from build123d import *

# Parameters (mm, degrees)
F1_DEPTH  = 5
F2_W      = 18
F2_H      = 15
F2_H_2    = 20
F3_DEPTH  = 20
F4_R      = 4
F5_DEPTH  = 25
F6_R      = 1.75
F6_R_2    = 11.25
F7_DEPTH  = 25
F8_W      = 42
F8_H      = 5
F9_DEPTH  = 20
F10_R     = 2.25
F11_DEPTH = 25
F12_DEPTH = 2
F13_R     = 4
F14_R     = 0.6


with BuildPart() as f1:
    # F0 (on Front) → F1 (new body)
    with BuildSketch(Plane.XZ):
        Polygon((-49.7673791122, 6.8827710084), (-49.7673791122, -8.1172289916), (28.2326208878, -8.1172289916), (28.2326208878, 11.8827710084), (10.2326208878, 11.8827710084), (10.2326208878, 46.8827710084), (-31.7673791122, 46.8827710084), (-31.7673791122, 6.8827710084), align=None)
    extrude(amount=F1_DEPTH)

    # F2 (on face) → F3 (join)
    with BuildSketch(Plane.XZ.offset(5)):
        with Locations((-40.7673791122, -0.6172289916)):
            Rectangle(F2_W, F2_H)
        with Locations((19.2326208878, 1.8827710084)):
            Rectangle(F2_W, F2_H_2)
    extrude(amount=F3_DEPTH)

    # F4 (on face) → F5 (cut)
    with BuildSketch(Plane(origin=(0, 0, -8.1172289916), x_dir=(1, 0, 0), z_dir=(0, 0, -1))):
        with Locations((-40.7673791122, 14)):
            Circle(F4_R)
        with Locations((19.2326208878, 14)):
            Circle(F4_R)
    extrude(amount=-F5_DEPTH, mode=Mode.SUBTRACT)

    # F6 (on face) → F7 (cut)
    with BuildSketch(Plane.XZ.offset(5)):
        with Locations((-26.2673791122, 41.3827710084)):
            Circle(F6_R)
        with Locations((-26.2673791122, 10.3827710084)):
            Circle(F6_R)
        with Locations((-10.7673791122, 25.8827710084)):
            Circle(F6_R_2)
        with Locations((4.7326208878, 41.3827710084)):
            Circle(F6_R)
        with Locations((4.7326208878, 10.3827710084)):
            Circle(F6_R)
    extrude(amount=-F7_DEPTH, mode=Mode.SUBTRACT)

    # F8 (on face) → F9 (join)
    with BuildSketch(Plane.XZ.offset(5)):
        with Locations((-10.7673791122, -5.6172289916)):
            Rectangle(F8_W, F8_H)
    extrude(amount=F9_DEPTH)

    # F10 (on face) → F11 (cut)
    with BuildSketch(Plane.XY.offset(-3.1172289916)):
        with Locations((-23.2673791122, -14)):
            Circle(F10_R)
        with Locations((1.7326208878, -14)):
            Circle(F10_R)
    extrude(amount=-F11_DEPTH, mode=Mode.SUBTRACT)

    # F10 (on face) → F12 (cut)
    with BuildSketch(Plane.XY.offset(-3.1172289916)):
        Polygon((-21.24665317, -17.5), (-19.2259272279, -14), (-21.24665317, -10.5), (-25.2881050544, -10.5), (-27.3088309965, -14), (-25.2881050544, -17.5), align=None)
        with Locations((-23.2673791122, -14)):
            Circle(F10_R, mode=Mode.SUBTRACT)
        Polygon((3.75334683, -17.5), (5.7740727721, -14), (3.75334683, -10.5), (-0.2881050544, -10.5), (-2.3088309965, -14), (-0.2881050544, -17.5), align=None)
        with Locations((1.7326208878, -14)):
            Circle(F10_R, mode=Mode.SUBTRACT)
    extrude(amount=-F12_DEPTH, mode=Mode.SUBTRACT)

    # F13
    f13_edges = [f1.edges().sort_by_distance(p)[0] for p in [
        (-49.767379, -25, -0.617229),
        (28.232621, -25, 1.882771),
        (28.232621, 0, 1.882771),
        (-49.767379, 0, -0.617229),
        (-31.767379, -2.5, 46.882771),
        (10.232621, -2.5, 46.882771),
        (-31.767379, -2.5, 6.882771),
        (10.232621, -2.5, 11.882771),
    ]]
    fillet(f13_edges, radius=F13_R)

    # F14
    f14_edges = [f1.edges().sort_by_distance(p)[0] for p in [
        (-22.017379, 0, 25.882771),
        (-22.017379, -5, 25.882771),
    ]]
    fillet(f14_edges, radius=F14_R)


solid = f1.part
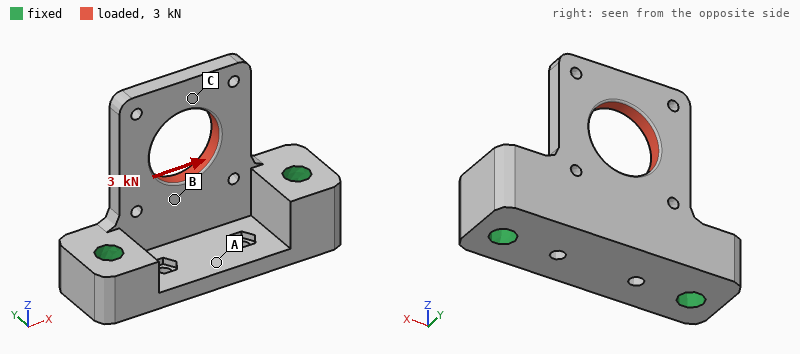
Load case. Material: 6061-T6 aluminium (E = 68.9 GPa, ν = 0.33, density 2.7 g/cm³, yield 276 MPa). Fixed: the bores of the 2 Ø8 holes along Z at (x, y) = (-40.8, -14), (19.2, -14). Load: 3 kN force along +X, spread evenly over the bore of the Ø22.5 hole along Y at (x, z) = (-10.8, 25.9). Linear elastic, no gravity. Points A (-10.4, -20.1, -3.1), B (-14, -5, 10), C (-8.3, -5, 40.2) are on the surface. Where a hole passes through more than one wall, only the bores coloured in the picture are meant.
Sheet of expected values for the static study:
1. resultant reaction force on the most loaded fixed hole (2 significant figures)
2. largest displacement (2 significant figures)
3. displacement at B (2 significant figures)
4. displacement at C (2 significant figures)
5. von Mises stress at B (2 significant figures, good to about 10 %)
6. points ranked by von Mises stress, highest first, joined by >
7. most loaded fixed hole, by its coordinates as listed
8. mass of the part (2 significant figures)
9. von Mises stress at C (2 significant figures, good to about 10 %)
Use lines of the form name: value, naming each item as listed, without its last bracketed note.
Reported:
resultant reaction force on the most loaded fixed hole: 2.3 kN
largest displacement: 74 µm
displacement at B: 11 µm
displacement at C: 67 µm
von Mises stress at B: 37 MPa
points ranked by von Mises stress, highest first, joined by >: B > C > A
most loaded fixed hole, by its coordinates as listed: (19.2, -14)
mass of the part: 73 g
von Mises stress at C: 20 MPa
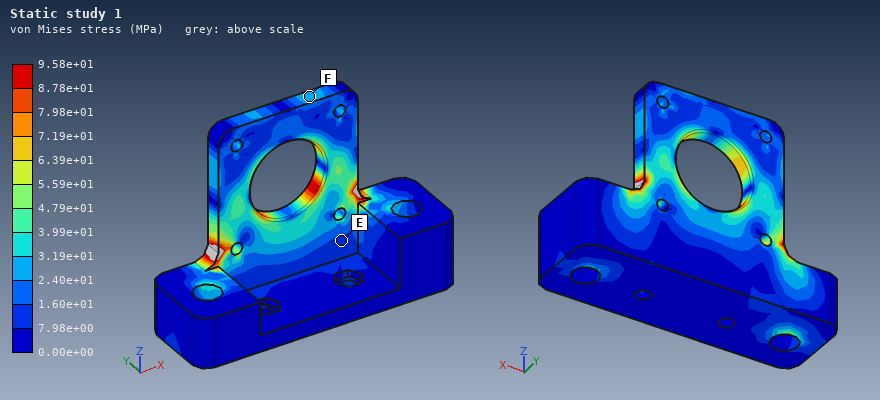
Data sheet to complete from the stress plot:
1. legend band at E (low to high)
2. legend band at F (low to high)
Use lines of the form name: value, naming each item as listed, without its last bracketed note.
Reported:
legend band at E: 7.98e+00 to 1.60e+01 MPa
legend band at F: 2.40e+01 to 3.19e+01 MPa
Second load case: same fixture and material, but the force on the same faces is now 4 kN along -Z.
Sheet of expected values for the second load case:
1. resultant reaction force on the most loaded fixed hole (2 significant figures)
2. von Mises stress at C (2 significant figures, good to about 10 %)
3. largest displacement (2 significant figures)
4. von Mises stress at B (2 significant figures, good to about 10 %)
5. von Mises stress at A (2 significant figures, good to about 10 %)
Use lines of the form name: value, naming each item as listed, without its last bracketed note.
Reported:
resultant reaction force on the most loaded fixed hole: 2.1 kN
von Mises stress at C: 13 MPa
largest displacement: 42 µm
von Mises stress at B: 16 MPa
von Mises stress at A: 5.6 MPa
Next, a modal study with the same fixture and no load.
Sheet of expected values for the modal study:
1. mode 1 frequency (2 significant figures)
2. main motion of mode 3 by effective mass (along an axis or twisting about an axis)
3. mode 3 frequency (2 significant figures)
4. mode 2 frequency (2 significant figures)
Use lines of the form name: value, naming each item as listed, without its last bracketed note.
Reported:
mode 1 frequency: 1900 Hz
main motion of mode 3 by effective mass: along X
mode 3 frequency: 8500 Hz
mode 2 frequency: 4700 Hz
